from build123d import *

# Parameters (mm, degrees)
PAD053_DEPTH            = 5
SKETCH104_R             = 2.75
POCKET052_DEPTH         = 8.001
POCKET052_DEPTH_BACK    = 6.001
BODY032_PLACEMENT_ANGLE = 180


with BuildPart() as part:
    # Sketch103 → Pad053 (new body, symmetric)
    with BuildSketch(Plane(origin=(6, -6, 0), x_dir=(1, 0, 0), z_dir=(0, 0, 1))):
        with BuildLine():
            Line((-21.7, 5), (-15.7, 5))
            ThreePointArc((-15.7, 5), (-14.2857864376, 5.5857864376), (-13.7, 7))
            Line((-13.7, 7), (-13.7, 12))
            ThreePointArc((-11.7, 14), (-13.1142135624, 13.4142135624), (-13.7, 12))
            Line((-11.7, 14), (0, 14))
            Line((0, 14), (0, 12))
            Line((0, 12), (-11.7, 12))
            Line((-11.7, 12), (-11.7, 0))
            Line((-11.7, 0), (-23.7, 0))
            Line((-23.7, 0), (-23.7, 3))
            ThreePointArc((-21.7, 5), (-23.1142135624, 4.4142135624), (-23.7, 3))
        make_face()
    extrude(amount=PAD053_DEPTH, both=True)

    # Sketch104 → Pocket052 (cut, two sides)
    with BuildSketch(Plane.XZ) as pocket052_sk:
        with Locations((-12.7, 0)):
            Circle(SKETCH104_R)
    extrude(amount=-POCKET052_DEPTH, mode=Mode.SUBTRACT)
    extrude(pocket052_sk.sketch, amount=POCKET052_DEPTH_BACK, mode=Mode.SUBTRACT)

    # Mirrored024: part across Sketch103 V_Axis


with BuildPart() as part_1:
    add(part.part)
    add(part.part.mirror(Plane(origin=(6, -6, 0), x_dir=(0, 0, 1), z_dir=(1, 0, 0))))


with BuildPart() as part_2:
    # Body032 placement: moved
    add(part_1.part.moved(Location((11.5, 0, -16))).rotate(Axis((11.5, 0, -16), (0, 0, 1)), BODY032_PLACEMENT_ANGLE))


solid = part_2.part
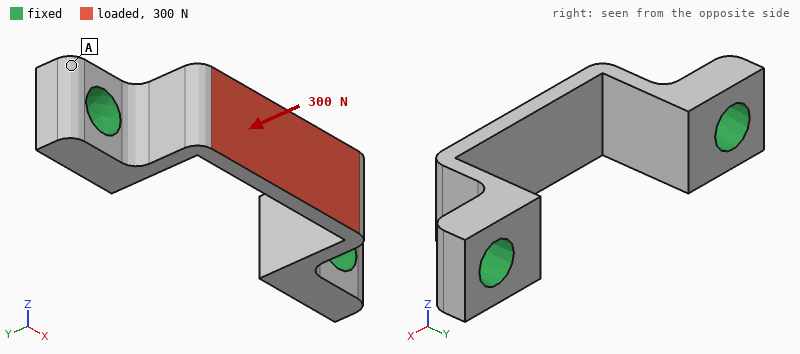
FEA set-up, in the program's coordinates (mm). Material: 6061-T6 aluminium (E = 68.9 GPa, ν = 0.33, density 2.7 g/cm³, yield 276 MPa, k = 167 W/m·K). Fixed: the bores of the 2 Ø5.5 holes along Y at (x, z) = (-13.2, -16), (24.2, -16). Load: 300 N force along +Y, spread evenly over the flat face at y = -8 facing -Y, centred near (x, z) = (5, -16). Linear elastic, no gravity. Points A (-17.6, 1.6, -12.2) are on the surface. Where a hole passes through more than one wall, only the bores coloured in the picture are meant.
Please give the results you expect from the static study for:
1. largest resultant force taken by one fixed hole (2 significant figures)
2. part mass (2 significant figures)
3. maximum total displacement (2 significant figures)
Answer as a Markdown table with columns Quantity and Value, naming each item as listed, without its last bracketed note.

| Quantity | Value |
|---|---|
| largest resultant force taken by one fixed hole | 190 N |
| part mass | 4.8 g |
| maximum total displacement | 45 µm |
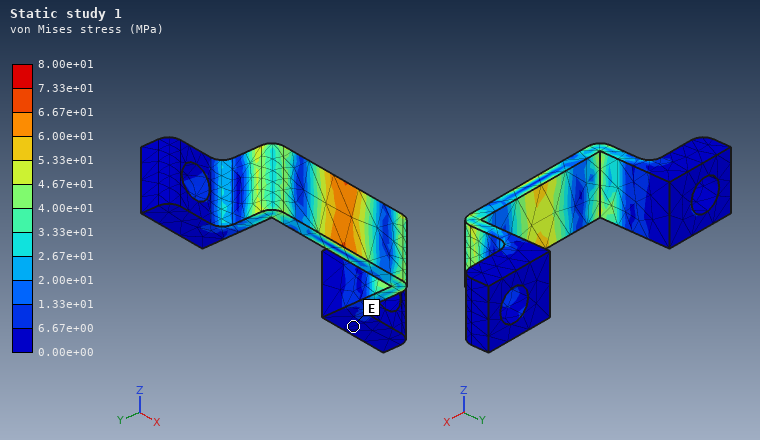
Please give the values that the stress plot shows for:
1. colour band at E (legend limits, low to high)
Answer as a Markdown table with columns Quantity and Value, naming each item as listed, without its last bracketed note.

| Quantity | Value |
|---|---|
| colour band at E | 0.00e+00 to 6.67e+00 MPa |
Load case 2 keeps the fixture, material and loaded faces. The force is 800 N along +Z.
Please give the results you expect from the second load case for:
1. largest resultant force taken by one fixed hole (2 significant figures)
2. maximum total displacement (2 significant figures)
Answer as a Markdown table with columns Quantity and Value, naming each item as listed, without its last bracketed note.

| Quantity | Value |
|---|---|
| largest resultant force taken by one fixed hole | 400 N |
| maximum total displacement | 67 µm |
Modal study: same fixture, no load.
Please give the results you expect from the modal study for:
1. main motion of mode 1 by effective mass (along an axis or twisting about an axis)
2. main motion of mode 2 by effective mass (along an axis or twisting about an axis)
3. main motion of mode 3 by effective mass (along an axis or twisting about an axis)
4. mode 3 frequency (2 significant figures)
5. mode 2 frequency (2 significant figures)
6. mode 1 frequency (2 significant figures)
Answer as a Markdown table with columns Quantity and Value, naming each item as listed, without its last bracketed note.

| Quantity | Value |
|---|---|
| main motion of mode 1 by effective mass | along X |
| main motion of mode 2 by effective mass | along Y |
| main motion of mode 3 by effective mass | along Z |
| mode 3 frequency | 17 kHz |
| mode 2 frequency | 13 kHz |
| mode 1 frequency | 12 kHz |
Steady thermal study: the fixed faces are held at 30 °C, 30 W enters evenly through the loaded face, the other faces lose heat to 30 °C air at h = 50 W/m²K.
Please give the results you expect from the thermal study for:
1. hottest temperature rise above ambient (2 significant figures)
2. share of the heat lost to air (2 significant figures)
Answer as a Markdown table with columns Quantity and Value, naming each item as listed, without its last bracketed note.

| Quantity | Value |
|---|---|
| hottest temperature rise above ambient | 69 K |
| share of the heat lost to air | 5.3 % |
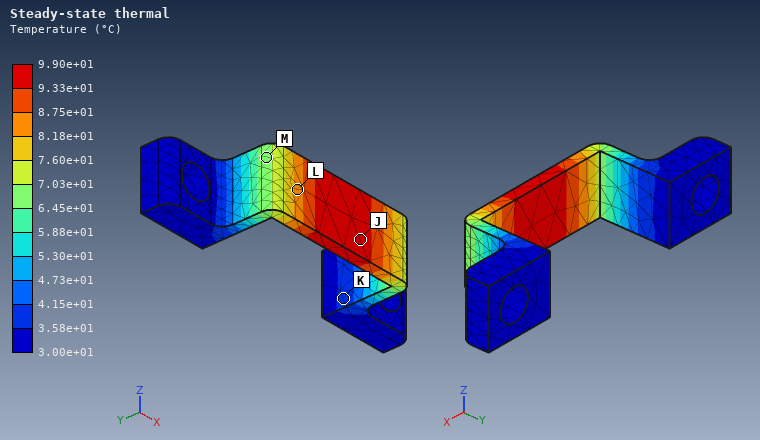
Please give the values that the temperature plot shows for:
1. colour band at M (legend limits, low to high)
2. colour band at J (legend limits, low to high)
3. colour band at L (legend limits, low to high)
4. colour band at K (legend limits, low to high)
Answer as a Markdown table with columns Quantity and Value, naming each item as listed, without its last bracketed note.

| Quantity | Value |
|---|---|
| colour band at M | 6.45e+01 to 7.03e+01 °C |
| colour band at J | 9.33e+01 to 9.90e+01 °C |
| colour band at L | 8.18e+01 to 8.75e+01 °C |
| colour band at K | 3.58e+01 to 4.15e+01 °C |
